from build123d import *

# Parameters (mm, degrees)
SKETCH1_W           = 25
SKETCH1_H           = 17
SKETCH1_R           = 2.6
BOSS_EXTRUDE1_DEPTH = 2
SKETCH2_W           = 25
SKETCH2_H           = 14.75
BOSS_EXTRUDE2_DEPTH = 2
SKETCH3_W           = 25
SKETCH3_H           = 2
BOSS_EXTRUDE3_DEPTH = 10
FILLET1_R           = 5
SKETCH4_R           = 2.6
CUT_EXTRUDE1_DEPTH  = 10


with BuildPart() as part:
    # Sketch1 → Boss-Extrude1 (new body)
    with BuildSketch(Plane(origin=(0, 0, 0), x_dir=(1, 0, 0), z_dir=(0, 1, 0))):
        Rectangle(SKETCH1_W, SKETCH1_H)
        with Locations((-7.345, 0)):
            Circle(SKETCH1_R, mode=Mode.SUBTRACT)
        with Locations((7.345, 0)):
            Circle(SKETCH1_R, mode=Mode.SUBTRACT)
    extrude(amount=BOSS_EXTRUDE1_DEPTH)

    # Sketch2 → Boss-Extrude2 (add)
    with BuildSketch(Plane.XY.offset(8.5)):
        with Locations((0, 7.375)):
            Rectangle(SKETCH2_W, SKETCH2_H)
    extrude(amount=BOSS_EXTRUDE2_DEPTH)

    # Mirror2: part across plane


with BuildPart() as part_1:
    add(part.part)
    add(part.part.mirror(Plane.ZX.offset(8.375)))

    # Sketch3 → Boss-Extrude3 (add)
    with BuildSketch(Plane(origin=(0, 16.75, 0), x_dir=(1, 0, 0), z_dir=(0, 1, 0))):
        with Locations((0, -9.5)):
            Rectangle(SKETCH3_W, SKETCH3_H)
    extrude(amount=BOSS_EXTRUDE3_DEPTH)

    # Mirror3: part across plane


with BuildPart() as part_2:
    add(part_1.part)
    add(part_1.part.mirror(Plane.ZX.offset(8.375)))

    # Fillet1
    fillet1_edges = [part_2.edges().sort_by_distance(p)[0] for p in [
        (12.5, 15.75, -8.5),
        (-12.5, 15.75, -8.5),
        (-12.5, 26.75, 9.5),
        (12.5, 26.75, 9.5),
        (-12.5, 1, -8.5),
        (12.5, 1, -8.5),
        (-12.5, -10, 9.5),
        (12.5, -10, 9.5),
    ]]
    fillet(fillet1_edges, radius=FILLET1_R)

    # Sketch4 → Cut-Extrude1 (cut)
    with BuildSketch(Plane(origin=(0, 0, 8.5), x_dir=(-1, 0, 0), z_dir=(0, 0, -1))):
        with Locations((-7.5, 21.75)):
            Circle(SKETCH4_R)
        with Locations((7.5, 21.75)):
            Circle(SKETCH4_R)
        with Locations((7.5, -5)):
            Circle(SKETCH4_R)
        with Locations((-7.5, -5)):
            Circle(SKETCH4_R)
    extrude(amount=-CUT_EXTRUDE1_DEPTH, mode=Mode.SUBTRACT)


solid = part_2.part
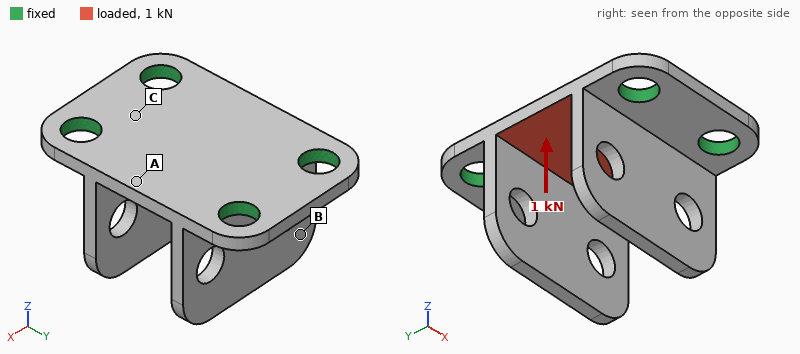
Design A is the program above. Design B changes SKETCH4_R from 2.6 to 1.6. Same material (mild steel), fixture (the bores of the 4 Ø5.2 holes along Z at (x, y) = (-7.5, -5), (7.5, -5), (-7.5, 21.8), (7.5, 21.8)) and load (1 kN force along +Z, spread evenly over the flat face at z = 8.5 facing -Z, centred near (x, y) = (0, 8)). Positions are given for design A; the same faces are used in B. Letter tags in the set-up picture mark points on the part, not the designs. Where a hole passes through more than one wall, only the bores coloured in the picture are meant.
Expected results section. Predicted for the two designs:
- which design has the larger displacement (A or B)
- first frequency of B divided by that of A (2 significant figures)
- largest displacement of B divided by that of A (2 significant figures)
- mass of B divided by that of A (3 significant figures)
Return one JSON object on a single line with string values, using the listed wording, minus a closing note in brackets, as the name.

{"which design has the larger displacement": "B", "first frequency of B divided by that of A": "0.96", "largest displacement of B divided by that of A": "1.3", "mass of B divided by that of A": "1.03"}
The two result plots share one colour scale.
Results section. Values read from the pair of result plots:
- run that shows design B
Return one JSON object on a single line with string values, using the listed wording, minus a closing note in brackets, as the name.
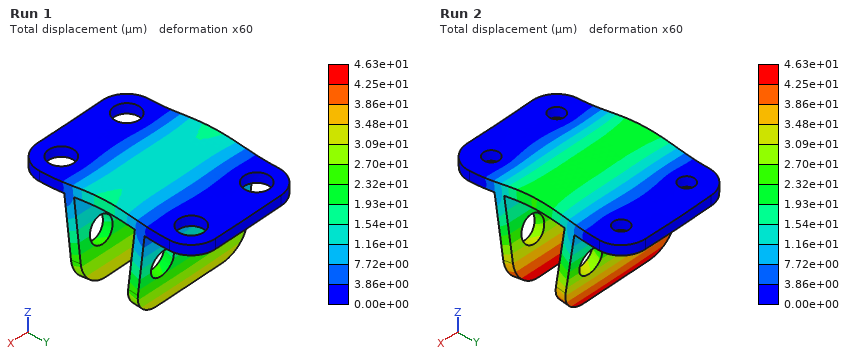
{"run that shows design B": "Run 2"}
